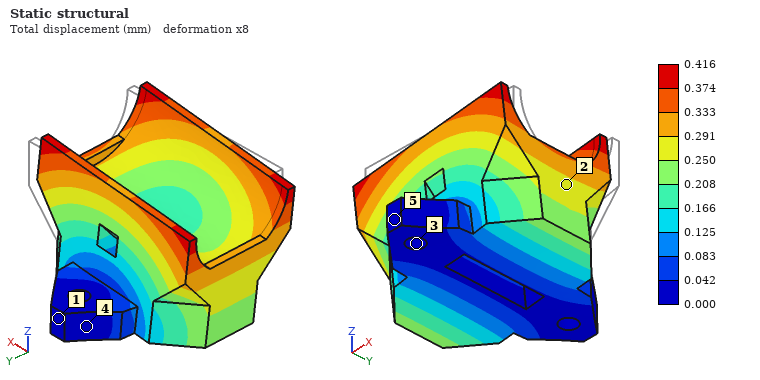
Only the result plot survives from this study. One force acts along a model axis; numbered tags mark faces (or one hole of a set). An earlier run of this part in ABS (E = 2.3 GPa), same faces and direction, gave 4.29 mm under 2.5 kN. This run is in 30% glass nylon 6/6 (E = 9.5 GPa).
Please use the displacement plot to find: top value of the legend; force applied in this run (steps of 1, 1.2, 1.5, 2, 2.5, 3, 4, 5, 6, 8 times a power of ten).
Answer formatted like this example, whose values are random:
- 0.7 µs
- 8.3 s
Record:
- 0.416 mm
- 1 kN
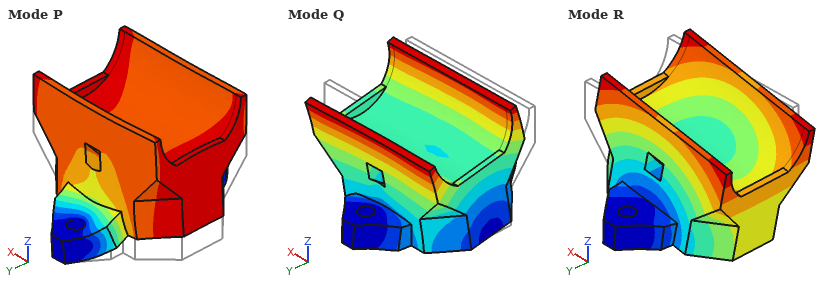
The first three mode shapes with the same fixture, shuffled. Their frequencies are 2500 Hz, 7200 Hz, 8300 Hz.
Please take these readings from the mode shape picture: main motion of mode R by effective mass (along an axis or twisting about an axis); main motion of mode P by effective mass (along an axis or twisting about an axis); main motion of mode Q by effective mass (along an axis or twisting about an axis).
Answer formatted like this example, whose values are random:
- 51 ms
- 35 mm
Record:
- along X
- along Z
- along Y
